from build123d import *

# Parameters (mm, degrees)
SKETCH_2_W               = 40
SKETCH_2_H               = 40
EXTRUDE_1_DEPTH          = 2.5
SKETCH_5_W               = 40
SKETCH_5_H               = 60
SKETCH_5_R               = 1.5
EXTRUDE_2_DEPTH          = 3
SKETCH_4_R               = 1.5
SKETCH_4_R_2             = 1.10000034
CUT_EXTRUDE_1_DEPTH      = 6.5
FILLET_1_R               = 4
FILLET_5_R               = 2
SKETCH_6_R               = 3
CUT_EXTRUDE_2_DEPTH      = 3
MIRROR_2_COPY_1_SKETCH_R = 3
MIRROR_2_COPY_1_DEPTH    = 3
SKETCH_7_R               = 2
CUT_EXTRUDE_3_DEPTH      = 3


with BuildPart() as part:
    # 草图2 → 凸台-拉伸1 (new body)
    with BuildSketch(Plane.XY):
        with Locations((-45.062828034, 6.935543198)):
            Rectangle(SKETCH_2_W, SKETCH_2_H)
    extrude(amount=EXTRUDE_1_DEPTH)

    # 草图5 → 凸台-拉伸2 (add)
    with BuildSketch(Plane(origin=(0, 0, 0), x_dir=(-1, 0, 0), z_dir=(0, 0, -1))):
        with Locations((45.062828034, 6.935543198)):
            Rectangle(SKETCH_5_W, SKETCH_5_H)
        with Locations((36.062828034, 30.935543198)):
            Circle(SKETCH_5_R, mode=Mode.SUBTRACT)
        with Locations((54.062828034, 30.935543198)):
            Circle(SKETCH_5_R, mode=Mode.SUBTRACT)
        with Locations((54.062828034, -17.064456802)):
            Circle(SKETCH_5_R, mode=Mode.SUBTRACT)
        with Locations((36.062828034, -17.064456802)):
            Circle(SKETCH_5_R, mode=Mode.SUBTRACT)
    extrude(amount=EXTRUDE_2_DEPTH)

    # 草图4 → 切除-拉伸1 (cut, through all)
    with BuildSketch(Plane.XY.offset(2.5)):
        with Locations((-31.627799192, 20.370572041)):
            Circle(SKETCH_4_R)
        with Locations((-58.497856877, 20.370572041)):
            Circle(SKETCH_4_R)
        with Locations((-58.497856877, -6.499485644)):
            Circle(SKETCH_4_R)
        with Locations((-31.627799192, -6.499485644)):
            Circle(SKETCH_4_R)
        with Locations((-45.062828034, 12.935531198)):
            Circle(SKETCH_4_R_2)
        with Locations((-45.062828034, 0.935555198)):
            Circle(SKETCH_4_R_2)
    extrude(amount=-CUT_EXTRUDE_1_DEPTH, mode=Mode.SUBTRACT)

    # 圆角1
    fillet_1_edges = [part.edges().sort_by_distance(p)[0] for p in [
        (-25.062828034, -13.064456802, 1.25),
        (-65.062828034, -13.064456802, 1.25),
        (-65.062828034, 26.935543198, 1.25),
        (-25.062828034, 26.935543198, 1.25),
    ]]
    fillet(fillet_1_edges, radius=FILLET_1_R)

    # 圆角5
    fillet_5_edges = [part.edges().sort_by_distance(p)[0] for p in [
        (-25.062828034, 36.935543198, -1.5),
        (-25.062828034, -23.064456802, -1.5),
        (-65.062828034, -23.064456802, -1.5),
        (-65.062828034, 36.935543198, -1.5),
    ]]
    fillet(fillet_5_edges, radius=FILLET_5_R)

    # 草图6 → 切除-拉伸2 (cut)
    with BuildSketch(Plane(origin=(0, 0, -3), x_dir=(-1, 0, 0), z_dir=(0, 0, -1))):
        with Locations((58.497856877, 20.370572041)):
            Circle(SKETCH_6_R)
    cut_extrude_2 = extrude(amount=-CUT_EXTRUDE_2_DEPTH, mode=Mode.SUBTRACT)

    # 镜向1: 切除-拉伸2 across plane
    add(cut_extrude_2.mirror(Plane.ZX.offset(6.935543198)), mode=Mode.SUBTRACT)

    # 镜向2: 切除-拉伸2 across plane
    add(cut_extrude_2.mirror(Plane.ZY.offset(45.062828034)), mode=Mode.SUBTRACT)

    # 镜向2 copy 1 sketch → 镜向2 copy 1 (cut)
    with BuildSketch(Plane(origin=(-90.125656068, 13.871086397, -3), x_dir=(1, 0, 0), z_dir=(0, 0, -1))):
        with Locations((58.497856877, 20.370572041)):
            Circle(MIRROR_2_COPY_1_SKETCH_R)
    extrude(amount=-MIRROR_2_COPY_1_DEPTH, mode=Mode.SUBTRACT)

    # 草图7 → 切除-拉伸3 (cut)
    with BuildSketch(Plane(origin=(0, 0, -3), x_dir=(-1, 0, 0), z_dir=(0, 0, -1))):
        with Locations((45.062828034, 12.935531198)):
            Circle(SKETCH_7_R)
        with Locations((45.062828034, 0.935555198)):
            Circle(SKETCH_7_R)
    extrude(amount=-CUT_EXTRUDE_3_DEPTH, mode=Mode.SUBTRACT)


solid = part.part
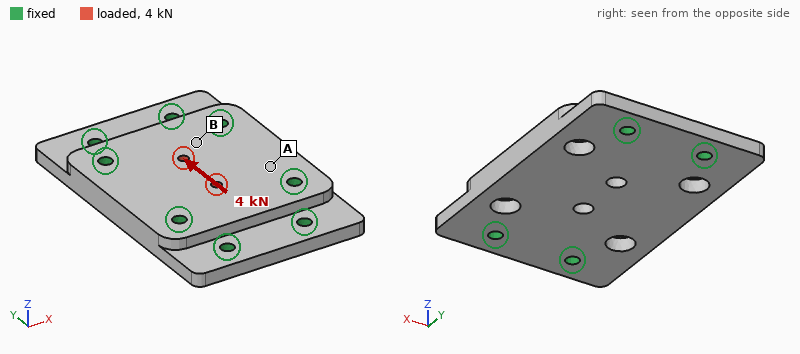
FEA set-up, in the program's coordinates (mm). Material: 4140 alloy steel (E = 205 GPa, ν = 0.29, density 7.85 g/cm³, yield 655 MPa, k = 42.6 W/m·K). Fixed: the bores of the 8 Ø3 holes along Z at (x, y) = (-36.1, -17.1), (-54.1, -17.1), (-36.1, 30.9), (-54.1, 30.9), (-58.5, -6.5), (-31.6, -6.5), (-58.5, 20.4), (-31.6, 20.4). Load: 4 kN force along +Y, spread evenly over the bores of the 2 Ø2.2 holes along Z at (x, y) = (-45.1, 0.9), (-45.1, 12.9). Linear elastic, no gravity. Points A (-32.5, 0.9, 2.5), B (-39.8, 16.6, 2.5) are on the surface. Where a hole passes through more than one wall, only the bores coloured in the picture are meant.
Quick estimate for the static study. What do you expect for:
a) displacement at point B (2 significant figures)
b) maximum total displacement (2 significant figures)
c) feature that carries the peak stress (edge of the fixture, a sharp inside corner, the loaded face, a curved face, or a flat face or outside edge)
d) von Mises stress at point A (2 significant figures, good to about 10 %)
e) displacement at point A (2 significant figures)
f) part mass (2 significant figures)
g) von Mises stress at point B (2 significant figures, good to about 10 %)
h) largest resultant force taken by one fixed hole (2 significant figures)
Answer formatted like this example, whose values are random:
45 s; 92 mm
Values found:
1.1 µm; 3.4 µm; the loaded face; 12 MPa; 0.50 µm; 83 g; 24 MPa; 560 N
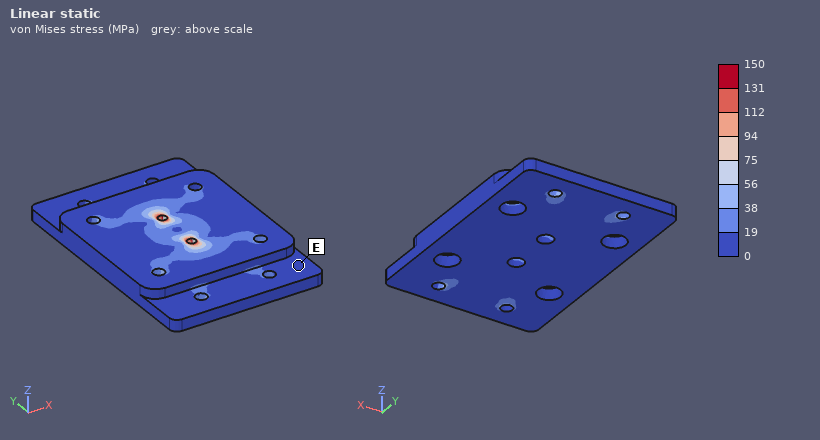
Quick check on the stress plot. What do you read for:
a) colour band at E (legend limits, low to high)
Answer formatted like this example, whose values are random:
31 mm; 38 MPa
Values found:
0 to 19 MPa
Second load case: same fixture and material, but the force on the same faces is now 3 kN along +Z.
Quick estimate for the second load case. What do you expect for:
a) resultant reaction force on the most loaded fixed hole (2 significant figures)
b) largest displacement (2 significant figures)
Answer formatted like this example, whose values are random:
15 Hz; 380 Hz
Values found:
1.0 kN; 14 µm
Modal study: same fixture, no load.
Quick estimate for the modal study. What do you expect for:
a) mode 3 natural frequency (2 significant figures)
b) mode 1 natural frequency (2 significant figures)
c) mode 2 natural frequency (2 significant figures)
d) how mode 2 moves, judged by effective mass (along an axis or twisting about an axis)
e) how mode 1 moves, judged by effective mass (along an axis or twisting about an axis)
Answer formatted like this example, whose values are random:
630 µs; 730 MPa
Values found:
29 kHz; 20 kHz; 26 kHz; twisting about Y; along Z
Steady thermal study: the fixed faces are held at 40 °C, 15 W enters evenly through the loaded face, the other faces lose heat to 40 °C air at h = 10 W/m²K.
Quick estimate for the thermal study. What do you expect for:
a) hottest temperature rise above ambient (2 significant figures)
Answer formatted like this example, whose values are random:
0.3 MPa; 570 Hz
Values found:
30 K
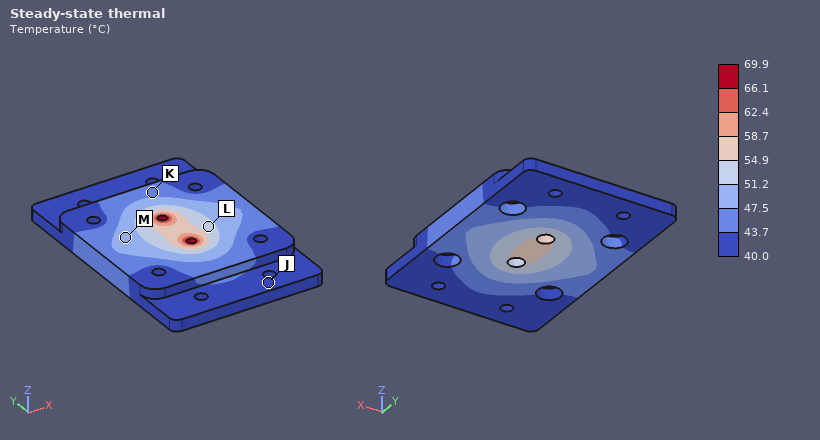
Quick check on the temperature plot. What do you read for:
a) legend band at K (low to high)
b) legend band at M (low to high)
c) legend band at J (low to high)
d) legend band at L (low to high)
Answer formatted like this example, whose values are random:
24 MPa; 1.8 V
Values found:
43.7 to 47.5 °C; 47.5 to 51.2 °C; 40.0 to 43.7 °C; 51.2 to 54.9 °C
